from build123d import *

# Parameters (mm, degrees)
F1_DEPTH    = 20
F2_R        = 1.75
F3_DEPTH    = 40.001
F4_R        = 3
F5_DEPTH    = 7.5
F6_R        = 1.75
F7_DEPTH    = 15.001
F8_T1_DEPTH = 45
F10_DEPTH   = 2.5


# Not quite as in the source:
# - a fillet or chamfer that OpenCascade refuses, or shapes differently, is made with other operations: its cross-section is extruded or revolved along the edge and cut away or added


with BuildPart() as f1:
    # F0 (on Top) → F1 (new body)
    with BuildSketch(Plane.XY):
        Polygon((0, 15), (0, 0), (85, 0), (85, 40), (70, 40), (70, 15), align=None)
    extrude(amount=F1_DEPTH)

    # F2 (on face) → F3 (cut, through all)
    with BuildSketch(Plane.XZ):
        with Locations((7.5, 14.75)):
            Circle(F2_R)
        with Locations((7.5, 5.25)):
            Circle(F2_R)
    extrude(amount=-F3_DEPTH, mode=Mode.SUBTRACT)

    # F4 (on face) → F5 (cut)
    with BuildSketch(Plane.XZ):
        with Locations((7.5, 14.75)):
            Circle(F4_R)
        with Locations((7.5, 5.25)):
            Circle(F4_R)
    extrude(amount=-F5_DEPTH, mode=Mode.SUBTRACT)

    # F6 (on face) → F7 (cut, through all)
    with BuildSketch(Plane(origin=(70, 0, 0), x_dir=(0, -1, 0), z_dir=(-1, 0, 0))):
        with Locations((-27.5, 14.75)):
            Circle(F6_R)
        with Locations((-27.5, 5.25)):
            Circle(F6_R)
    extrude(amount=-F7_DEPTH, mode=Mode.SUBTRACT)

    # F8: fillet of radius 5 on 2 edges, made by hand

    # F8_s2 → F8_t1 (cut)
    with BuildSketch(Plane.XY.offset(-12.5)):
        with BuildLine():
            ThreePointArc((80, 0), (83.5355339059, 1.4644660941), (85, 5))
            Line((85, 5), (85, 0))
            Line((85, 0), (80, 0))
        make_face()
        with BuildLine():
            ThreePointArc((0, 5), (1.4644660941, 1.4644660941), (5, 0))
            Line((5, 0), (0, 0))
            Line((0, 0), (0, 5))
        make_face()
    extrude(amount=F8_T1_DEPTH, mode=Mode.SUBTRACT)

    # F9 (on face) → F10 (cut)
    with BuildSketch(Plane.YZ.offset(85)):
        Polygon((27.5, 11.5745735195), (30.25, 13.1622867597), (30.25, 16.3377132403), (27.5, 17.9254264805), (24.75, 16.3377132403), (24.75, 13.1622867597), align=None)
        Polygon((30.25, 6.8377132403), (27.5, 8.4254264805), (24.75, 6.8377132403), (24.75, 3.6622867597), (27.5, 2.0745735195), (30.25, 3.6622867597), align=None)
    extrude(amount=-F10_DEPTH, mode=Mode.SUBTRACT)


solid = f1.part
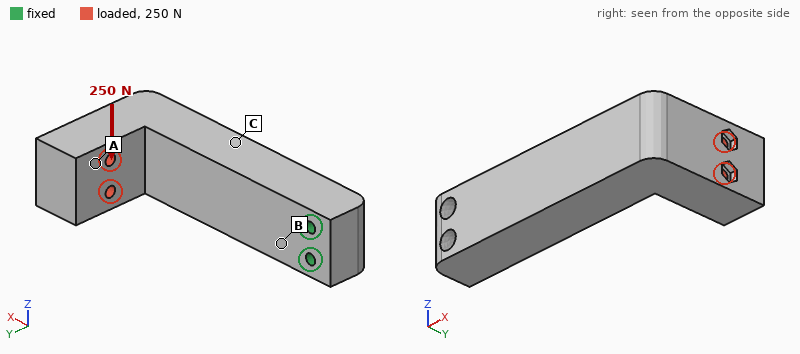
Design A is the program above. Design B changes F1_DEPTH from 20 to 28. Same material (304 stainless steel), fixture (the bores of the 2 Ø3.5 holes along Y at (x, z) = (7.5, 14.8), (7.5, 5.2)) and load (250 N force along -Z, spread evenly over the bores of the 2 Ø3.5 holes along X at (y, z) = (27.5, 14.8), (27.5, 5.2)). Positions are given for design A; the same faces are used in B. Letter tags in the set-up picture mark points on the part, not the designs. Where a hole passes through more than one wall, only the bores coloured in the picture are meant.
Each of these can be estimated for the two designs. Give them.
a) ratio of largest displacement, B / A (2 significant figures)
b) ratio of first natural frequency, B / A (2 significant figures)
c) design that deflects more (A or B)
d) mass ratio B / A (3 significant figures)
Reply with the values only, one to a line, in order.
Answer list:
0.62
0.92
A
1.41
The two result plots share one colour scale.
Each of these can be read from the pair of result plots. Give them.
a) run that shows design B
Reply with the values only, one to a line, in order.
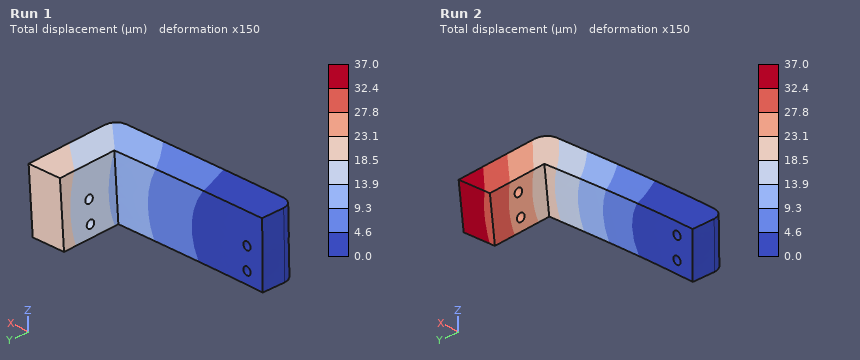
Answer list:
Run 1
